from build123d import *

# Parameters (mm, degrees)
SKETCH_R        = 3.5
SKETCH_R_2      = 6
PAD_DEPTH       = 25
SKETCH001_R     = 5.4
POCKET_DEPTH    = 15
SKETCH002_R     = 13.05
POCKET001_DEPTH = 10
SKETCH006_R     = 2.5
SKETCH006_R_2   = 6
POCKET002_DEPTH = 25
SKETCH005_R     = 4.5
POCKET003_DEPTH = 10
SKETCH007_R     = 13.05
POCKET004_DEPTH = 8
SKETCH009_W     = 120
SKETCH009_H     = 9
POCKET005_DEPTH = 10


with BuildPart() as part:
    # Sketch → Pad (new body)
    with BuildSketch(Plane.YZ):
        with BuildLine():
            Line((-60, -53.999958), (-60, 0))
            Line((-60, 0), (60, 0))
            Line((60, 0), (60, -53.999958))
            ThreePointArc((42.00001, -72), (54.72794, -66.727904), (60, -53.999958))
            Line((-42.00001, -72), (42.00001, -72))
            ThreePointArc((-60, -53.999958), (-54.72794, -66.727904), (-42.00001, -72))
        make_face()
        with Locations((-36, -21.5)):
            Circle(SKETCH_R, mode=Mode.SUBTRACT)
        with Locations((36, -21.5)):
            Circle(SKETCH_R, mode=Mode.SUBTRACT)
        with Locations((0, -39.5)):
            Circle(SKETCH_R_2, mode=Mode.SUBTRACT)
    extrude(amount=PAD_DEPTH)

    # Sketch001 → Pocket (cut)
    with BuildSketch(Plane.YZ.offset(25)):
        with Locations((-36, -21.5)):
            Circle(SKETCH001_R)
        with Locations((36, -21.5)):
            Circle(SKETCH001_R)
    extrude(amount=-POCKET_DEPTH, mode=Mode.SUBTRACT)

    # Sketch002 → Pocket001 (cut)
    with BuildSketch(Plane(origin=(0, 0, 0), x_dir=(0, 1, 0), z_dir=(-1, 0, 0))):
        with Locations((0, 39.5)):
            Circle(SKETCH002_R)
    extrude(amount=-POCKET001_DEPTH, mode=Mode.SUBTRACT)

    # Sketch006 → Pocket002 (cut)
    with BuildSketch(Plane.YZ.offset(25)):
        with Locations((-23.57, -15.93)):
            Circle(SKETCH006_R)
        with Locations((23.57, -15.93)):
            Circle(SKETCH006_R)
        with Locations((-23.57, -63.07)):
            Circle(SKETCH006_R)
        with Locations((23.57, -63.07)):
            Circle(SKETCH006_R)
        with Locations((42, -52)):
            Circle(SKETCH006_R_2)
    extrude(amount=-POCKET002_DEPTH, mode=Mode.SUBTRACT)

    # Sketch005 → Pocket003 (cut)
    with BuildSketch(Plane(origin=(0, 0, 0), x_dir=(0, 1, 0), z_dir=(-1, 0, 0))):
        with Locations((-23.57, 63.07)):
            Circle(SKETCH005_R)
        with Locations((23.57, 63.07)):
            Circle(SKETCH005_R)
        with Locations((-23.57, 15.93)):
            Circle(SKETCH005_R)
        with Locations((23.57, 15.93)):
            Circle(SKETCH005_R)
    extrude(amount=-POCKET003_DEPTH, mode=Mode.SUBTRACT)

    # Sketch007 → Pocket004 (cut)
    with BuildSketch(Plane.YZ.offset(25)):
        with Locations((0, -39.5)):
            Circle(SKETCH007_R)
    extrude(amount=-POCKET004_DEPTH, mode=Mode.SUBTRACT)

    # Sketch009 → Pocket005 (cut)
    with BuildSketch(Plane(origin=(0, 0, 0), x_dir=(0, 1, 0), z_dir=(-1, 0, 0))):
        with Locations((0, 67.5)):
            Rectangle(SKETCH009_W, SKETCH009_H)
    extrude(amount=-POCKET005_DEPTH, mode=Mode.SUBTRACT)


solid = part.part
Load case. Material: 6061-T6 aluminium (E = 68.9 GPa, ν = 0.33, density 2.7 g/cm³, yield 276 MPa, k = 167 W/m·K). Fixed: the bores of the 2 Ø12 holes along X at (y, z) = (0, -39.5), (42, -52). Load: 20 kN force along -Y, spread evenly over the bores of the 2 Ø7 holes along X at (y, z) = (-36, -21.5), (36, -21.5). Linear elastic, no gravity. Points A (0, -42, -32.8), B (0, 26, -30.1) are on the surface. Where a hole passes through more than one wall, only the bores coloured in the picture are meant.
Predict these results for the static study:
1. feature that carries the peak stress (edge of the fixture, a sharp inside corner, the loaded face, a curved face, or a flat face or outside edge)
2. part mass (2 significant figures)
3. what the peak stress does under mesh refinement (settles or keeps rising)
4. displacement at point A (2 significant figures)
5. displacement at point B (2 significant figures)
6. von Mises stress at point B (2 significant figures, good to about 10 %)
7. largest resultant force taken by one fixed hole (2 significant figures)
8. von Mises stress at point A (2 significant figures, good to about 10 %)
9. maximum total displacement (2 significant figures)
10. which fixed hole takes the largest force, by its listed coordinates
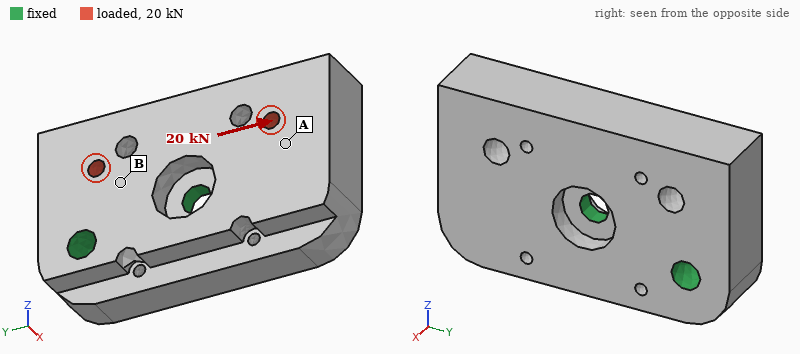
edge of the fixture
490 g
keeps rising
51 µm
14 µm
33 MPa
15 kN
17 MPa
82 µm
(0, -39.5)
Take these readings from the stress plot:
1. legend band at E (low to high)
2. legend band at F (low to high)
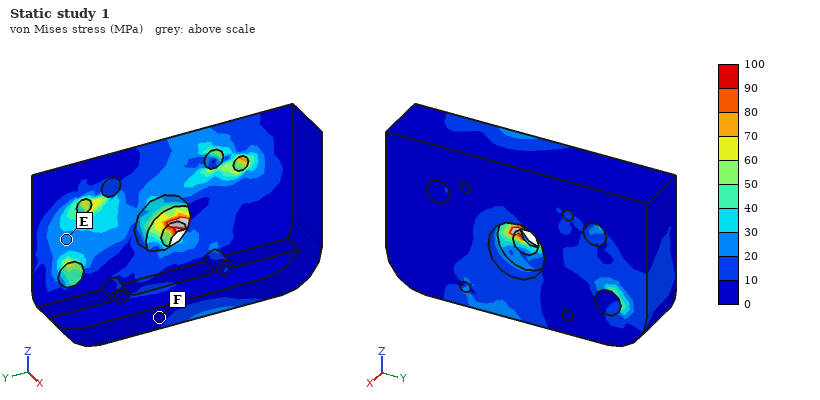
20 to 30 MPa
0 to 10 MPa
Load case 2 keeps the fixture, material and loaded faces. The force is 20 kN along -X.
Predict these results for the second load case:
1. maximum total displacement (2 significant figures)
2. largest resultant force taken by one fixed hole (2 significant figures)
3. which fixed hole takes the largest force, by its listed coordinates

0.32 mm
18 kN
(0, -39.5)
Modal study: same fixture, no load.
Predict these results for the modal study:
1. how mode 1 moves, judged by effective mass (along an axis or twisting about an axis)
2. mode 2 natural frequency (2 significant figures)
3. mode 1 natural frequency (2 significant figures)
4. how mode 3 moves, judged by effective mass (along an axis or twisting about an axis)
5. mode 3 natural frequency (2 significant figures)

along X
4000 Hz
2700 Hz
along Z
5000 Hz
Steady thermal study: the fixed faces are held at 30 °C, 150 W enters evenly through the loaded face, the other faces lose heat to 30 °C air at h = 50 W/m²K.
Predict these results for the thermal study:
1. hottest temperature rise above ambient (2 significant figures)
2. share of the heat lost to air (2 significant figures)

29 K
11 %
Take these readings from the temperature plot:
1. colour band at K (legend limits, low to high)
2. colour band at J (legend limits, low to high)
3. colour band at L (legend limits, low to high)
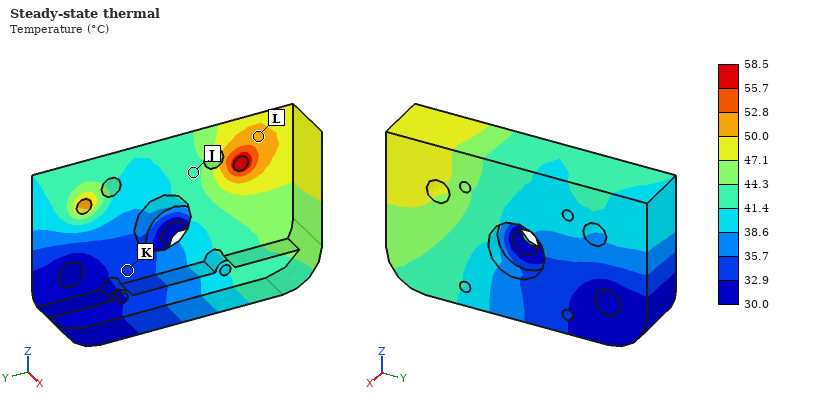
32.9 to 35.7 °C
41.4 to 44.3 °C
50.0 to 52.8 °C
